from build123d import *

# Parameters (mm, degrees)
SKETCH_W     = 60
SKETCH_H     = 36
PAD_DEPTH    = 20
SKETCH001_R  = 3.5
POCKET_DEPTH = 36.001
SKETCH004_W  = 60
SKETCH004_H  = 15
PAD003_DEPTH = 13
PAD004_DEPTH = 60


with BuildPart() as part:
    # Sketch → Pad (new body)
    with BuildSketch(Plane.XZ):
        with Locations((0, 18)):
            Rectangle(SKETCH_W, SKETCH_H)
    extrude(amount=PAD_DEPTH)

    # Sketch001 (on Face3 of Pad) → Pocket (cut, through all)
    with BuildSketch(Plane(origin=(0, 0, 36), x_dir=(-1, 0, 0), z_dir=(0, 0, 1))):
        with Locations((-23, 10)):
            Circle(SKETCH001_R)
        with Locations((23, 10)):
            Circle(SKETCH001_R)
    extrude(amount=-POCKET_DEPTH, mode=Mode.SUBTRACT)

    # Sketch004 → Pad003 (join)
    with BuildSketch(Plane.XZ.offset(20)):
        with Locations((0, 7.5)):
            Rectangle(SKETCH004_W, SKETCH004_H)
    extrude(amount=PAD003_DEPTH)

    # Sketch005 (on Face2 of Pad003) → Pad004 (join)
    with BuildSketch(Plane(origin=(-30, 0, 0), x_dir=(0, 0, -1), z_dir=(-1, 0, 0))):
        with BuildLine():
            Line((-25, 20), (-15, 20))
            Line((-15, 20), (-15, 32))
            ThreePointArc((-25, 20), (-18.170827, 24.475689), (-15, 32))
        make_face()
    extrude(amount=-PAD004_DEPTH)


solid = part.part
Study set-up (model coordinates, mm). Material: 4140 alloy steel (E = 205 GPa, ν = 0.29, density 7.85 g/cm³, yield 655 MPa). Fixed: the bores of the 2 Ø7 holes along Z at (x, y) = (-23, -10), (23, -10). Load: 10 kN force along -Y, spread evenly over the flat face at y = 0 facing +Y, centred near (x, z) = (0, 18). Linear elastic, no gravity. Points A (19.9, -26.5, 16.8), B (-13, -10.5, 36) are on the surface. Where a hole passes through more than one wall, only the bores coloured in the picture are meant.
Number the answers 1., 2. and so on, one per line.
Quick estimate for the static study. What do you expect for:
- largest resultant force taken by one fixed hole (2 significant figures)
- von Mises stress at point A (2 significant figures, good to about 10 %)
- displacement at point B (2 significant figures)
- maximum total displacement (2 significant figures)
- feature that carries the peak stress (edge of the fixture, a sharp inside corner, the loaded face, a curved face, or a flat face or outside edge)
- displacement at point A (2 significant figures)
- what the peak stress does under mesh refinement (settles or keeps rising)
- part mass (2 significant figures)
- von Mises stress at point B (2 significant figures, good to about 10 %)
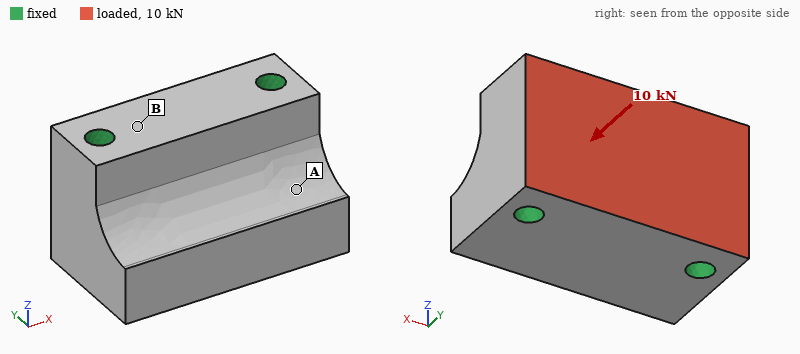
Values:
1. 5.0 kN
2. 3.1 MPa
3. 0.73 µm
4. 1.5 µm
5. edge of the fixture
6. 0.36 µm
7. keeps rising
8. 430 g
9. 7.8 MPa
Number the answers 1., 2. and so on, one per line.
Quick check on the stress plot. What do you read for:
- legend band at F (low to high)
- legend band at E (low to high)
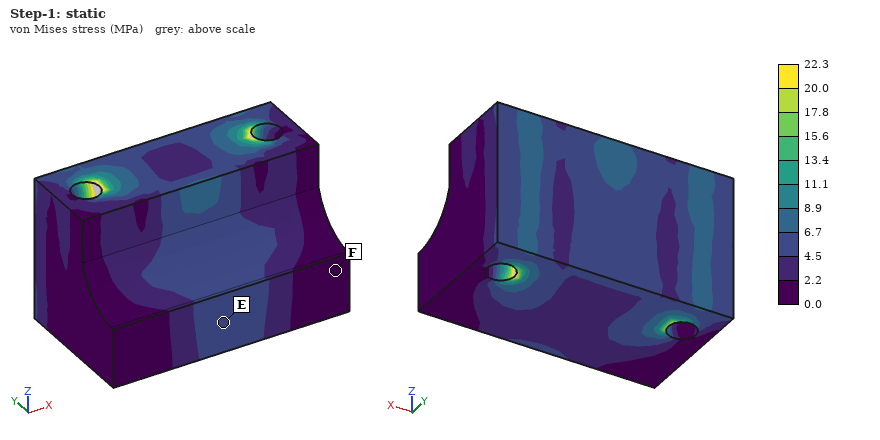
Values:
1. 0.0 to 2.2 MPa
2. 4.5 to 6.7 MPa
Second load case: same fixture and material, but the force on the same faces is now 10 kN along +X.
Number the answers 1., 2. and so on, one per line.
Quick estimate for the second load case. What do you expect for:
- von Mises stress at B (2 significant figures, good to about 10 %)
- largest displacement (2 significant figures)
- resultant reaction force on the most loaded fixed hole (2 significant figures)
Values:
1. 5.6 MPa
2. 1.1 µm
3. 5.3 kN
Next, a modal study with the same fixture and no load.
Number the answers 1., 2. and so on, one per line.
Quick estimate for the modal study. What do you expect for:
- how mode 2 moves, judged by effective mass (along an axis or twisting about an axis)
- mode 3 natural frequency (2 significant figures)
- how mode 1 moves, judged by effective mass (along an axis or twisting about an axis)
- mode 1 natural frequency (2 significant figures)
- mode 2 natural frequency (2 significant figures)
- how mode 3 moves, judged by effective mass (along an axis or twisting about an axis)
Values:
1. along Y
2. 31 kHz
3. along Z
4. 23 kHz
5. 26 kHz
6. along Z
